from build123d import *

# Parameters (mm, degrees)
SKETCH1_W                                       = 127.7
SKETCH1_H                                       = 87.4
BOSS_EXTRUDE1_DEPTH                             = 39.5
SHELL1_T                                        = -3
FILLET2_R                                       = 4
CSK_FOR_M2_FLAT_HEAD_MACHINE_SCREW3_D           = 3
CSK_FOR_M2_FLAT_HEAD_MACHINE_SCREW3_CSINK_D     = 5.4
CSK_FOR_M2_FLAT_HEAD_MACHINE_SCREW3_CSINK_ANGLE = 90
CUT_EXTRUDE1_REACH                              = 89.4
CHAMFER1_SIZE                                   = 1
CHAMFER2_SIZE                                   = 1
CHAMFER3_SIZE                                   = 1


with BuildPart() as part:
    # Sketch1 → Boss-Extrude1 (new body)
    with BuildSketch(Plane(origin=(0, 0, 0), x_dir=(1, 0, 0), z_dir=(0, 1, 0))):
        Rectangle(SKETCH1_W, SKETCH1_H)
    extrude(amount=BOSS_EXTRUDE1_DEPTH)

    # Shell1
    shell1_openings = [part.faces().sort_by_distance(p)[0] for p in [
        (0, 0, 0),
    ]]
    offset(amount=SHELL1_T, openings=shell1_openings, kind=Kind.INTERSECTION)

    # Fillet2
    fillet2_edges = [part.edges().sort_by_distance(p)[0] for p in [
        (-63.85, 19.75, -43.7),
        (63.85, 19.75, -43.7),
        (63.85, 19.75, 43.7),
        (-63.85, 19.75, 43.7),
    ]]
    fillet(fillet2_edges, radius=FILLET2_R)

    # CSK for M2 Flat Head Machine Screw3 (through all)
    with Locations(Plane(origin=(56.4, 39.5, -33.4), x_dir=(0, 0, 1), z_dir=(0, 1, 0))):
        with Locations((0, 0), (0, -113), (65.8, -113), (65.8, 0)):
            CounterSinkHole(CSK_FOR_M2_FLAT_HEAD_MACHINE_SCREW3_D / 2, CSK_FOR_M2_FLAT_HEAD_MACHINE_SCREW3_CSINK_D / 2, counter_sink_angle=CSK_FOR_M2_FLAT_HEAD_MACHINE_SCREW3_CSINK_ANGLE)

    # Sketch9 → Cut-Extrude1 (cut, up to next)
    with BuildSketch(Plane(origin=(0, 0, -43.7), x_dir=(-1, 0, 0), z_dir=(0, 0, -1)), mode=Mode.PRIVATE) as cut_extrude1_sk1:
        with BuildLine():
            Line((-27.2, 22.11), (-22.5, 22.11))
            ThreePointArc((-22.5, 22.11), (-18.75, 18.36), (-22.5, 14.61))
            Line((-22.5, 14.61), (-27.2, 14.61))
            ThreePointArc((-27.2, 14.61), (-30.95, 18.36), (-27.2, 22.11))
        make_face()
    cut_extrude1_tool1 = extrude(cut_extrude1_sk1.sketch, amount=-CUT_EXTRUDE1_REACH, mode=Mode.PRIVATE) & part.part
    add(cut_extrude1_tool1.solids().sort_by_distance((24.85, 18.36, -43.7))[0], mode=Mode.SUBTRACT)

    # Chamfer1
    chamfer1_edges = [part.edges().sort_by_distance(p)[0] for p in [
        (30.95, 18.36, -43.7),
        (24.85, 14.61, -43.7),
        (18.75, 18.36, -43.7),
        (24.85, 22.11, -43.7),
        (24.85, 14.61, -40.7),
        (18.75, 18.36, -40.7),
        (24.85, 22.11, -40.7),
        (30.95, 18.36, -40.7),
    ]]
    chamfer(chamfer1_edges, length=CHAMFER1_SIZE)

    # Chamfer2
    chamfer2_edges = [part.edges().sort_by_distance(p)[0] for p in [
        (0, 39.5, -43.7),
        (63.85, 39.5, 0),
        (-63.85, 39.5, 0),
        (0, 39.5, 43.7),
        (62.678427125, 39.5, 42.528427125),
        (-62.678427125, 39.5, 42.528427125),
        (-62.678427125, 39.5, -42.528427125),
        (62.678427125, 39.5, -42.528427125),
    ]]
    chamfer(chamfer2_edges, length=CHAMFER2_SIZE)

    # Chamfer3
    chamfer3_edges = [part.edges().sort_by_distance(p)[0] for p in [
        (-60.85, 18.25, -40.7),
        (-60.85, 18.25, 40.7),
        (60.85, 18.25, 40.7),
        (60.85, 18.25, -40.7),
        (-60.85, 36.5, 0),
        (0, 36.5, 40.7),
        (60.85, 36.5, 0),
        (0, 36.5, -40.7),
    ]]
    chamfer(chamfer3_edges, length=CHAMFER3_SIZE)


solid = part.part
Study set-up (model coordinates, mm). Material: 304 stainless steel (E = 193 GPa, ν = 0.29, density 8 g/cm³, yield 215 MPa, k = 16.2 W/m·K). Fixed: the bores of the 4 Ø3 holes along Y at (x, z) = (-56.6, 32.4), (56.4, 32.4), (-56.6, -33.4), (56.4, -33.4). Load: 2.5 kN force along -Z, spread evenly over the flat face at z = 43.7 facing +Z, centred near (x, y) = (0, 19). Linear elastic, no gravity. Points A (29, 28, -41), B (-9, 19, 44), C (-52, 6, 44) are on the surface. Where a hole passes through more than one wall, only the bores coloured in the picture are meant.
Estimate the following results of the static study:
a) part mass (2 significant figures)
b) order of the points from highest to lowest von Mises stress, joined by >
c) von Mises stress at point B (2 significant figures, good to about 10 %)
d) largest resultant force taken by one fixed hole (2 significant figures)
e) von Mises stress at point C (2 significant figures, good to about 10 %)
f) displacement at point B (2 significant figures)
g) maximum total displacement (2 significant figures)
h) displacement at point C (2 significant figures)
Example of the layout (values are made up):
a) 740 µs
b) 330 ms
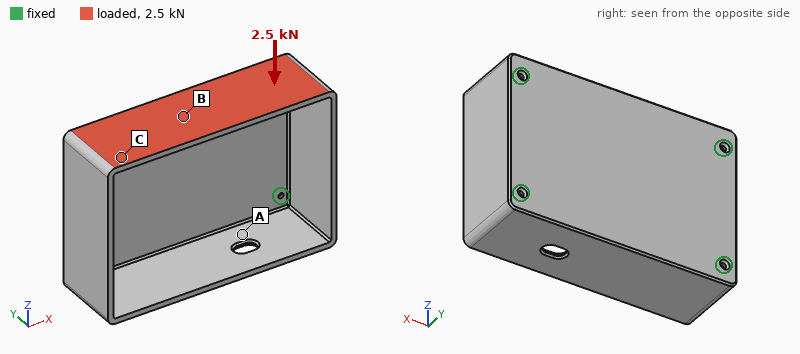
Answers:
a) 630 g
b) C > B > A
c) 42 MPa
d) 810 N
e) 96 MPa
f) 0.17 mm
g) 0.37 mm
h) 0.066 mm
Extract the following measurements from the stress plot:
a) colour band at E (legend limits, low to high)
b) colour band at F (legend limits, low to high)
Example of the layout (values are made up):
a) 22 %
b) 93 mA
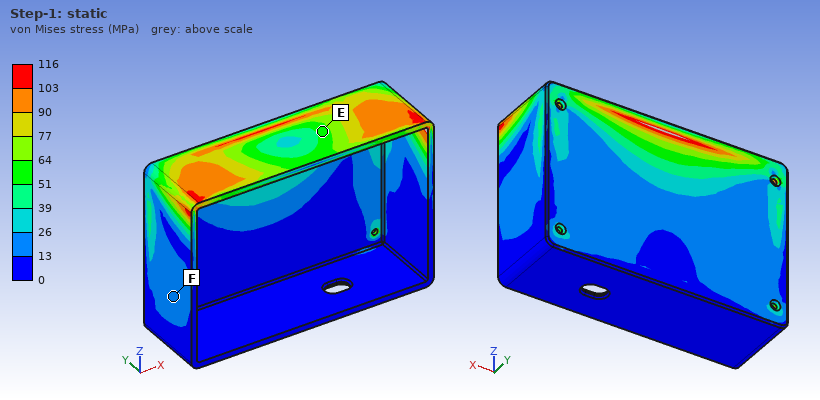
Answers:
a) 51 to 64 MPa
b) 13 to 26 MPa
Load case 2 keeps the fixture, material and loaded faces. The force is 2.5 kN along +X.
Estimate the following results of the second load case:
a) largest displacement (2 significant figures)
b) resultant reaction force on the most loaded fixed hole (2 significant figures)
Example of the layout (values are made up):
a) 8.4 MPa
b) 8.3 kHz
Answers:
a) 8.7 µm
b) 1.2 kN
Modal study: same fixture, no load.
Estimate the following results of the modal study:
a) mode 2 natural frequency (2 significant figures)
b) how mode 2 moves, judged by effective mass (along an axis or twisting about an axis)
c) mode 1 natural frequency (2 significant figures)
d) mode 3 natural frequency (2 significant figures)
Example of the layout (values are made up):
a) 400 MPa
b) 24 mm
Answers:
a) 1700 Hz
b) along Z
c) 1500 Hz
d) 2200 Hz
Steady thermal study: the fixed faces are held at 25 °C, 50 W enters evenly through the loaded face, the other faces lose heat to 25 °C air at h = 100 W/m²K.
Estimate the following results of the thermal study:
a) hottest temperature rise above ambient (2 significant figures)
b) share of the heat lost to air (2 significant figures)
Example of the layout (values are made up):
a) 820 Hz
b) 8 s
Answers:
a) 75 K
b) 93 %
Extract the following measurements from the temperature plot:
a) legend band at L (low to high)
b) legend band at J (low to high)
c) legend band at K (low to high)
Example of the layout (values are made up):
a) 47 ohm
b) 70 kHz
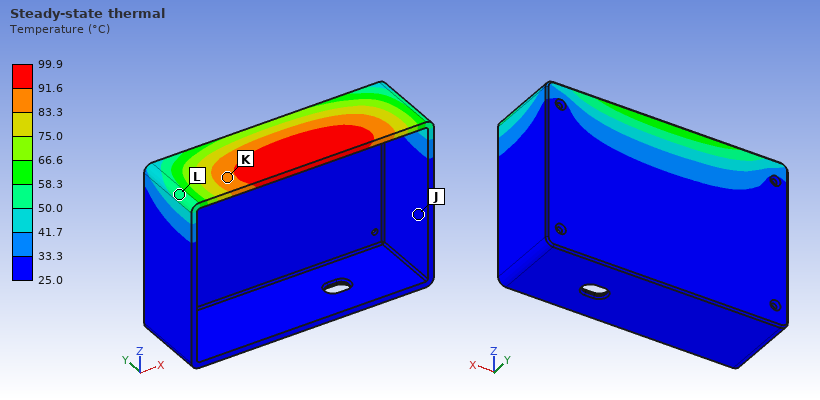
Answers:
a) 50.0 to 58.3 °C
b) 25.0 to 33.3 °C
c) 83.3 to 91.6 °C
